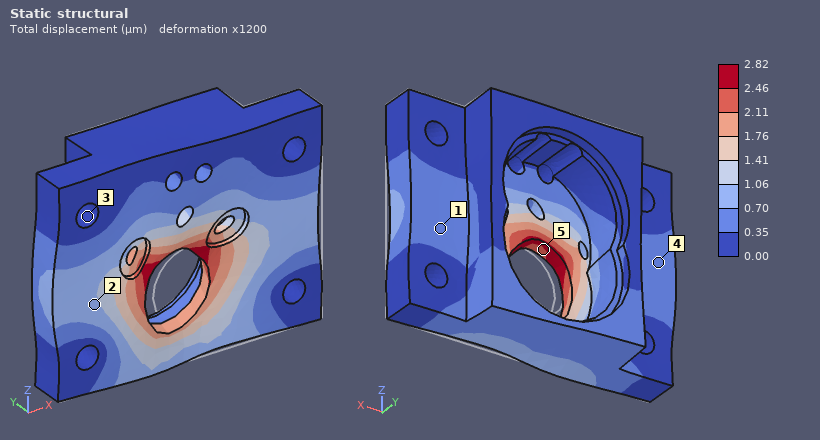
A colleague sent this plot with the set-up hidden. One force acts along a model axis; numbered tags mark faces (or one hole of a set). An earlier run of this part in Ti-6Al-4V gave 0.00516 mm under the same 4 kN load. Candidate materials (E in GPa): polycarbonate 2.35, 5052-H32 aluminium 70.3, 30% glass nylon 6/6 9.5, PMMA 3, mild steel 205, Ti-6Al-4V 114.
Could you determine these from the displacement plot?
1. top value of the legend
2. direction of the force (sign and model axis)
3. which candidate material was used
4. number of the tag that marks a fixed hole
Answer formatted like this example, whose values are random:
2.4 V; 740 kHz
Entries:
2.82 µm; -X; mild steel; 3
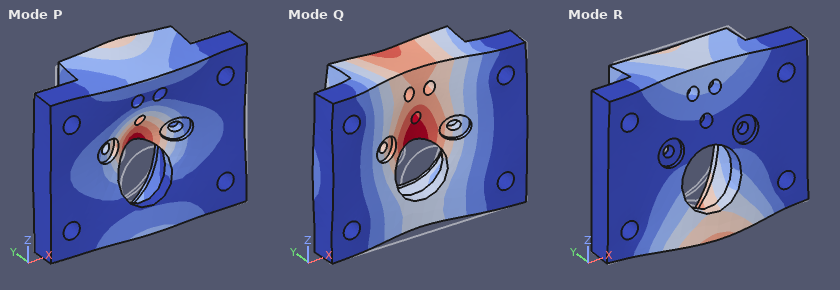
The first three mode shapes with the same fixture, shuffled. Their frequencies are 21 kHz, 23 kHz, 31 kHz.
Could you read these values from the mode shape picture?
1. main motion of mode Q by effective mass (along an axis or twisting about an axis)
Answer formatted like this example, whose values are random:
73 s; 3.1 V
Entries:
along Y
